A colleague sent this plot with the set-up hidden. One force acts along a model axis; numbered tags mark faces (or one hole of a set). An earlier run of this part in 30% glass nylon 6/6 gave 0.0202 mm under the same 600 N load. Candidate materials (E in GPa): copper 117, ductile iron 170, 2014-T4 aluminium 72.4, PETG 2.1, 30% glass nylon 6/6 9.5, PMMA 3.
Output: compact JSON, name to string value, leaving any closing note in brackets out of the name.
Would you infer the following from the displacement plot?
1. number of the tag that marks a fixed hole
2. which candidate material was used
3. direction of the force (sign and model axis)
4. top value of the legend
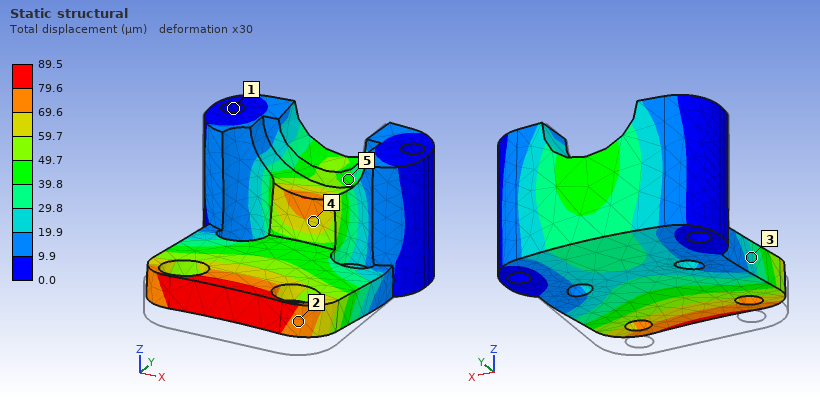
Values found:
{"number of the tag that marks a fixed hole": "1", "which candidate material was used": "PETG", "direction of the force": "+Y", "top value of the legend": "89.5 µm"}
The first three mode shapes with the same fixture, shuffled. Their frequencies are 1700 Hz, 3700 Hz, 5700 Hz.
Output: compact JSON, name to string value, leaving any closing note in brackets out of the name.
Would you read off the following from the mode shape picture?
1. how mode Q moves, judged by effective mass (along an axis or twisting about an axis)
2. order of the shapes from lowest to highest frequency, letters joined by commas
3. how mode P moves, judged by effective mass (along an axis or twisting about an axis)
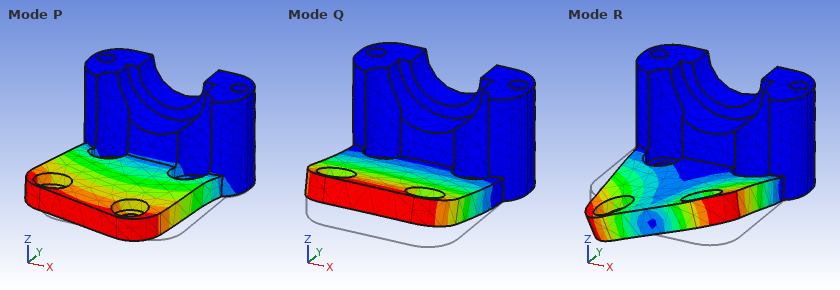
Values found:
{"how mode Q moves, judged by effective mass": "along Z", "order of the shapes from lowest to highest frequency, letters joined by commas": "Q, R, P", "how mode P moves, judged by effective mass": "along X"}
